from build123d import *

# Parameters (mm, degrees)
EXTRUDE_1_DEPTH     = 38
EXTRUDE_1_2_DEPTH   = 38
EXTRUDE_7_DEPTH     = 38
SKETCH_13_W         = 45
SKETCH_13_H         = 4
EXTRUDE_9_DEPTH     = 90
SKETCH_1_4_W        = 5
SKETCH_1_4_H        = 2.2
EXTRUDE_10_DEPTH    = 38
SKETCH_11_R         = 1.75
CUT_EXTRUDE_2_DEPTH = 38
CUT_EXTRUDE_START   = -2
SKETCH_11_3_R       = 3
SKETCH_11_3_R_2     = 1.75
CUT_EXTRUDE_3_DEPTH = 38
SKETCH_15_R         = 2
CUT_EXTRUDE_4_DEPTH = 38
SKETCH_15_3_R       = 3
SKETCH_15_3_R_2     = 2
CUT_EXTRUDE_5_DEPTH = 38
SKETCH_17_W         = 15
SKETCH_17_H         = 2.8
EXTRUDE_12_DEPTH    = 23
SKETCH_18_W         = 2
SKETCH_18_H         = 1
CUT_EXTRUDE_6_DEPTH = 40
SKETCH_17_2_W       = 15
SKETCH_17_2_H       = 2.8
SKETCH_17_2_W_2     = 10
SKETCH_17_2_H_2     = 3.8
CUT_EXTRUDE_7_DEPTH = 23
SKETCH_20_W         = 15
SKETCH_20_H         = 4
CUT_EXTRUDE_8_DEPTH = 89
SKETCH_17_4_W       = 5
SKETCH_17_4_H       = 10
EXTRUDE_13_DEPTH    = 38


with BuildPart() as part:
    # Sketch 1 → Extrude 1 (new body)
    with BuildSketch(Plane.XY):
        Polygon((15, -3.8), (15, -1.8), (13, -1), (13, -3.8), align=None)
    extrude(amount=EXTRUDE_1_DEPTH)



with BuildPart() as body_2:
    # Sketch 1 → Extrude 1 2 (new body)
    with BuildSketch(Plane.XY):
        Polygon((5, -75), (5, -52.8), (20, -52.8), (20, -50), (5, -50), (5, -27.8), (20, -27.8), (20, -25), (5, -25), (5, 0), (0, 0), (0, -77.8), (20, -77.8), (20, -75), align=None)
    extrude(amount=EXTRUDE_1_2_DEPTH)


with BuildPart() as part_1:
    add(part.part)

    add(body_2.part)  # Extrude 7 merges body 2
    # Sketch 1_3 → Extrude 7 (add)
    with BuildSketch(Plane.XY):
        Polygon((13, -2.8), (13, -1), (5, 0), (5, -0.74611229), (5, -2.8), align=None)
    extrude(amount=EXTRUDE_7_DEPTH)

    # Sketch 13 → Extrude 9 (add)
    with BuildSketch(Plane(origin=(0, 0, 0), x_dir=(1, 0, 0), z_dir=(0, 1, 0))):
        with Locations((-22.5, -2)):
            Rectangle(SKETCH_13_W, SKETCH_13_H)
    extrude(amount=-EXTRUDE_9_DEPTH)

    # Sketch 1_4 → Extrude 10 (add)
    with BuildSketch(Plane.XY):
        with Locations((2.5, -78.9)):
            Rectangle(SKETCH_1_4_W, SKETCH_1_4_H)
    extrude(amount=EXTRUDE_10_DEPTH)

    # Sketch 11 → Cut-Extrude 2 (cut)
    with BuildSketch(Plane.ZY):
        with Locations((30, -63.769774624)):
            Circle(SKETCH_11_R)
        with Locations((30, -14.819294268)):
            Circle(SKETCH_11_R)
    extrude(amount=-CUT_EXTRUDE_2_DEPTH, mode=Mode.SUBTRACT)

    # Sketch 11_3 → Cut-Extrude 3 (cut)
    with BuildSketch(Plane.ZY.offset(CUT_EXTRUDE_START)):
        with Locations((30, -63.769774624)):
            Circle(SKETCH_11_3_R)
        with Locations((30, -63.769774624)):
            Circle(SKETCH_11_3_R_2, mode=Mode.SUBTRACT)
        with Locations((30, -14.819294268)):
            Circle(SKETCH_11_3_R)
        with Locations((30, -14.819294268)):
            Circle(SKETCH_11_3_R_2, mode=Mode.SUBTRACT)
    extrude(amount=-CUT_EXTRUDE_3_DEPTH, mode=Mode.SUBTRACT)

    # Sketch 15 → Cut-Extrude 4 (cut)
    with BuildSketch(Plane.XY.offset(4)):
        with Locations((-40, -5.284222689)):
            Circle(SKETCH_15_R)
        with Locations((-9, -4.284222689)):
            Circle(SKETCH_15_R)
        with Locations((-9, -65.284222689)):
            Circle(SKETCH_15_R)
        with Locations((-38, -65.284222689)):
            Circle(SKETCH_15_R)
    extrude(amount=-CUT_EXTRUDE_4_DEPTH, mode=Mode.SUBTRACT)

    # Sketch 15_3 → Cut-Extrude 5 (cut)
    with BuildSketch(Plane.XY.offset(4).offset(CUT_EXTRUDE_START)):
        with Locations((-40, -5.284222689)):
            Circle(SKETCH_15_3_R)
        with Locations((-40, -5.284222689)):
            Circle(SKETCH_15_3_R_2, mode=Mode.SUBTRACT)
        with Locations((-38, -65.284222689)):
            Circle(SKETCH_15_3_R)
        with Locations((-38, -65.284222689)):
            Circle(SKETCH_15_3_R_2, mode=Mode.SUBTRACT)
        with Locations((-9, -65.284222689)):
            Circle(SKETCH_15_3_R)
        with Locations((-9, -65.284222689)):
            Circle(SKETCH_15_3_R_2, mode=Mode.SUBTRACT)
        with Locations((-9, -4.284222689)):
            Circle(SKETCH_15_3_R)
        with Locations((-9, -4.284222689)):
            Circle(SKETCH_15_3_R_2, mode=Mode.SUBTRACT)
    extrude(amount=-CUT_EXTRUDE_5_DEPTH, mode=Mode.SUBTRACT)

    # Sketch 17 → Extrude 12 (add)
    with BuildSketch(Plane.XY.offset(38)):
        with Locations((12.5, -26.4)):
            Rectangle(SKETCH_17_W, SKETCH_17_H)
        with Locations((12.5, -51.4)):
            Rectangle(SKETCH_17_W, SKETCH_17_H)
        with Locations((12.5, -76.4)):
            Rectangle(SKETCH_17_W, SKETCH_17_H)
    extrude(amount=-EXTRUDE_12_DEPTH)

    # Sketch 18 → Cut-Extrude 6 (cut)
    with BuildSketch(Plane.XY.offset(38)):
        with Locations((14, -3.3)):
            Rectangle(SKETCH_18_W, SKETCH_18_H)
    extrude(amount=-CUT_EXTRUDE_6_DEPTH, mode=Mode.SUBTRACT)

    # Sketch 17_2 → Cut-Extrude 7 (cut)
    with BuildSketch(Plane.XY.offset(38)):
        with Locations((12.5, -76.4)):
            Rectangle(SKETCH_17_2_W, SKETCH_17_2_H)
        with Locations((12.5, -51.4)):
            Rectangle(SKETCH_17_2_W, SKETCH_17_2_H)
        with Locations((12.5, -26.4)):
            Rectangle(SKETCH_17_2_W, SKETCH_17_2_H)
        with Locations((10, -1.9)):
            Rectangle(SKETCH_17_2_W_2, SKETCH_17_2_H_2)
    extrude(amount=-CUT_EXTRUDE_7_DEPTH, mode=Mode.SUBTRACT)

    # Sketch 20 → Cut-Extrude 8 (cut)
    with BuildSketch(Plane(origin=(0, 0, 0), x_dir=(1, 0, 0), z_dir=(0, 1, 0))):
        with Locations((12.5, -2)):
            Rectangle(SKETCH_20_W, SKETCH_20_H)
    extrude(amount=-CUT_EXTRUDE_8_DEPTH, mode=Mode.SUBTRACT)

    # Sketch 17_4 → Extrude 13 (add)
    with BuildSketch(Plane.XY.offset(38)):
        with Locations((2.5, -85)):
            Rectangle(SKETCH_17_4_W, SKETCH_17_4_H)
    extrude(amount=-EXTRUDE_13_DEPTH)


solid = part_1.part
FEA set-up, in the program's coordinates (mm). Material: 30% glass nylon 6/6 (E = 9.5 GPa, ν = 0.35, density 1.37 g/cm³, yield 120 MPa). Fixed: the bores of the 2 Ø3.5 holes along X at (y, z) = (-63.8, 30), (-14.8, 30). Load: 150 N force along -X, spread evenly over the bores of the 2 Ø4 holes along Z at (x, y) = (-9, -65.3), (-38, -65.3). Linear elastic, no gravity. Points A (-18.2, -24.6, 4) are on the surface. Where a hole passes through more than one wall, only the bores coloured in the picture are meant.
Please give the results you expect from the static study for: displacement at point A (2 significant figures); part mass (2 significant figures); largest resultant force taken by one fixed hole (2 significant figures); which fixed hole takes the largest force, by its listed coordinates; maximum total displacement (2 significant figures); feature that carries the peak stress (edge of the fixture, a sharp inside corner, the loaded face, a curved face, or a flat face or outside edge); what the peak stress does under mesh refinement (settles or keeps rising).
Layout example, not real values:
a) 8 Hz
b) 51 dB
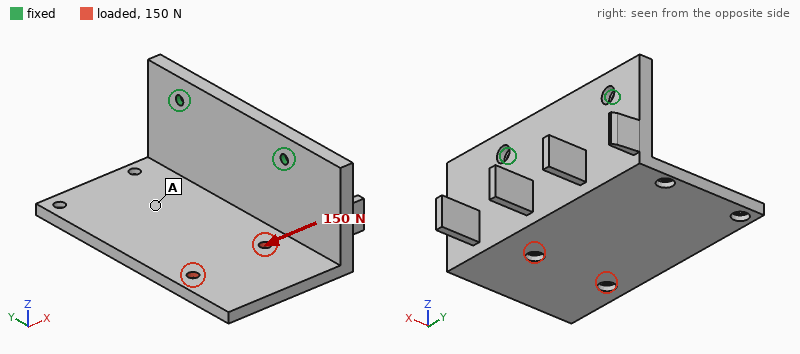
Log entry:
a) 0.58 mm
b) 47 g
c) 150 N
d) (-63.8, 30)
e) 1.4 mm
f) edge of the fixture
g) keeps rising
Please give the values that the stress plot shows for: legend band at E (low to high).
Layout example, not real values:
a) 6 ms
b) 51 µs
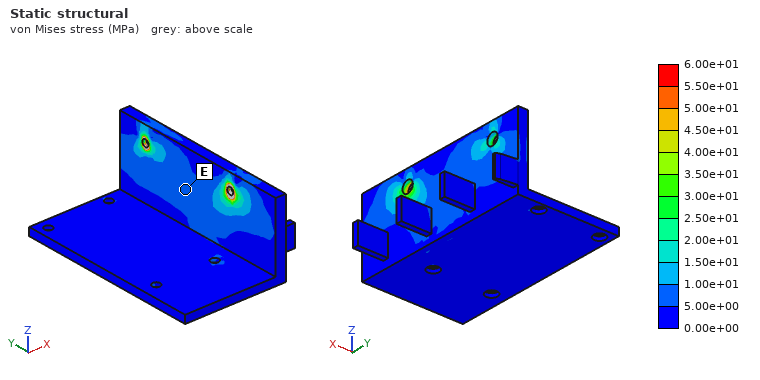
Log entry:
a) 5.00e+00 to 1.00e+01 MPa
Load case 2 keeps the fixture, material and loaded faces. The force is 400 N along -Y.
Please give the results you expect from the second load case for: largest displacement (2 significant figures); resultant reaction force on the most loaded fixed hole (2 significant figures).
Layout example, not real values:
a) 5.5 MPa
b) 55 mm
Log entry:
a) 1.1 mm
b) 360 N
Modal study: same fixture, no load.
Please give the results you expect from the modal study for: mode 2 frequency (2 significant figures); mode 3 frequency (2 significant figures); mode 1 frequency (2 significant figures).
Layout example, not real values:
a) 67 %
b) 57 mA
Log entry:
a) 660 Hz
b) 970 Hz
c) 330 Hz
